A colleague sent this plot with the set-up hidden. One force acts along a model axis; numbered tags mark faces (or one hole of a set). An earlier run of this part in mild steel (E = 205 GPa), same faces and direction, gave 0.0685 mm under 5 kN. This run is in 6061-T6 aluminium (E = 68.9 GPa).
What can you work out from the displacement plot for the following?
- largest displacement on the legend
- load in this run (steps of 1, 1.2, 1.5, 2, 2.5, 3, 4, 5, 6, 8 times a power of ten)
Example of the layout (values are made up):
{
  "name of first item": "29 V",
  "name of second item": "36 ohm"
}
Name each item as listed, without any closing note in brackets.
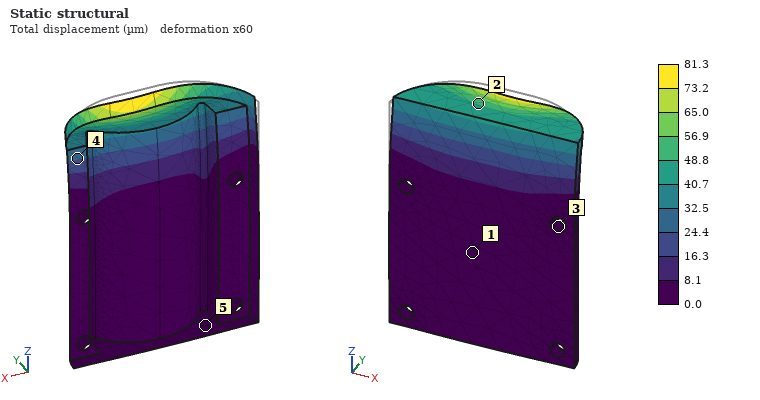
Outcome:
{
  "largest displacement on the legend": "81.3 µm",
  "load in this run": "2 kN"
}
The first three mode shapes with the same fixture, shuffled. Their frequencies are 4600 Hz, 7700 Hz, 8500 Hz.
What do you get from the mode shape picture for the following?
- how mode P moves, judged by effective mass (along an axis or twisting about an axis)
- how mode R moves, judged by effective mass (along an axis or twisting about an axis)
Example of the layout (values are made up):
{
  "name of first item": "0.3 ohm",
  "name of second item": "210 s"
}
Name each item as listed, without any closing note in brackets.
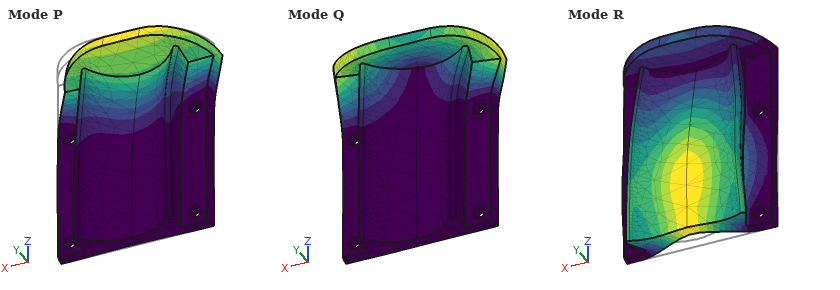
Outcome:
{
  "how mode P moves, judged by effective mass": "along Y",
  "how mode R moves, judged by effective mass": "along Y"
}
